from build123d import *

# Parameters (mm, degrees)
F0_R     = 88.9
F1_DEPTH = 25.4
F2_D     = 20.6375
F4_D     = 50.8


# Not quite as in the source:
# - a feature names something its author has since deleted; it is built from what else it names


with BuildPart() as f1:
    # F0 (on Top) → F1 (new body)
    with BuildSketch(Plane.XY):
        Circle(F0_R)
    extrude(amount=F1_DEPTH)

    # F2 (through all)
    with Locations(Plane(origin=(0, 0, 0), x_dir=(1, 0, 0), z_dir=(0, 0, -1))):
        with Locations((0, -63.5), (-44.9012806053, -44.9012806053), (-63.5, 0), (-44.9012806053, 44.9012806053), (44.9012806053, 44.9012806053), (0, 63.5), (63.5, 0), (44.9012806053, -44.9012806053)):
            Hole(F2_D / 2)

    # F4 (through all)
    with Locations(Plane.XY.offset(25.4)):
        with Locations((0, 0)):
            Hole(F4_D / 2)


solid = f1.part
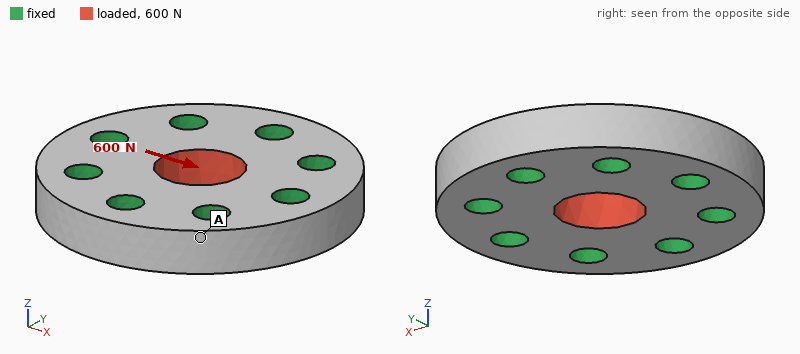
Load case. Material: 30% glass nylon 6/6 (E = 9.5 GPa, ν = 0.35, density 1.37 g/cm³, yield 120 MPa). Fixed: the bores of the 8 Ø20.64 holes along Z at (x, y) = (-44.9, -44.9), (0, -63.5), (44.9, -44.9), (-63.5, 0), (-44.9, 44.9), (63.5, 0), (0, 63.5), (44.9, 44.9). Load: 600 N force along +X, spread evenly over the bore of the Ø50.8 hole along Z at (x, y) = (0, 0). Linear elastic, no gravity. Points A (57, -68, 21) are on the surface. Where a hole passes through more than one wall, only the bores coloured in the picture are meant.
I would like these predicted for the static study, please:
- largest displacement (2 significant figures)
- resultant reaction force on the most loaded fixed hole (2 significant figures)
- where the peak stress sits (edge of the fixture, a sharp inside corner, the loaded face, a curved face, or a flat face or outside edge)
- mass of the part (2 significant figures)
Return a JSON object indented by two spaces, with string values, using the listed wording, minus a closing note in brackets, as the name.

{
  "largest displacement": "0.53 µm",
  "resultant reaction force on the most loaded fixed hole": "130 N",
  "where the peak stress sits": "the loaded face",
  "mass of the part": "700 g"
}
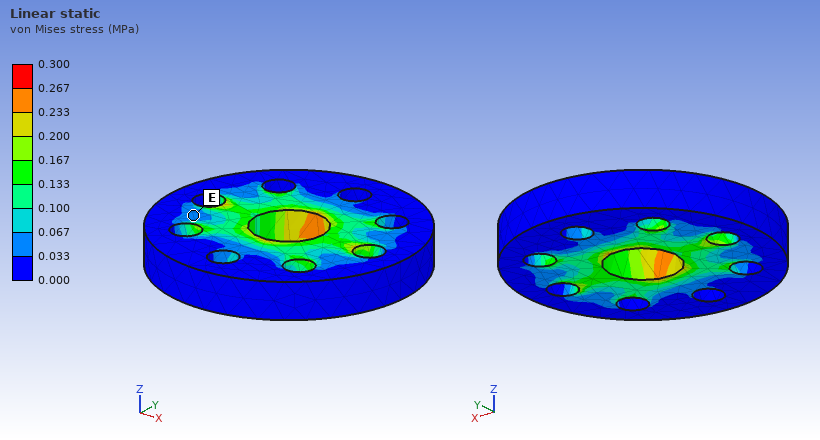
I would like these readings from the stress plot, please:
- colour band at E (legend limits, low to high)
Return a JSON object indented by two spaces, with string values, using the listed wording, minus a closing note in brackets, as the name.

{
  "colour band at E": "0.033 to 0.067 MPa"
}
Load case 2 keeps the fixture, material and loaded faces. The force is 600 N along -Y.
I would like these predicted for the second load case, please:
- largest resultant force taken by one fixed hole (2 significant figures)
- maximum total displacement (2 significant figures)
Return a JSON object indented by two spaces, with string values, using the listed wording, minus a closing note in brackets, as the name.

{
  "largest resultant force taken by one fixed hole": "130 N",
  "maximum total displacement": "0.54 µm"
}
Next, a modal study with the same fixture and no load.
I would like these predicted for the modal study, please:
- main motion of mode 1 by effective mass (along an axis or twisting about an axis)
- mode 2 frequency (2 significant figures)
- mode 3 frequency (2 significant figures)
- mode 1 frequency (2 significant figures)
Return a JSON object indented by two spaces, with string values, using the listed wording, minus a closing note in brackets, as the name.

{
  "main motion of mode 1 by effective mass": "along Z",
  "mode 2 frequency": "11 kHz",
  "mode 3 frequency": "11 kHz",
  "mode 1 frequency": "9400 Hz"
}
